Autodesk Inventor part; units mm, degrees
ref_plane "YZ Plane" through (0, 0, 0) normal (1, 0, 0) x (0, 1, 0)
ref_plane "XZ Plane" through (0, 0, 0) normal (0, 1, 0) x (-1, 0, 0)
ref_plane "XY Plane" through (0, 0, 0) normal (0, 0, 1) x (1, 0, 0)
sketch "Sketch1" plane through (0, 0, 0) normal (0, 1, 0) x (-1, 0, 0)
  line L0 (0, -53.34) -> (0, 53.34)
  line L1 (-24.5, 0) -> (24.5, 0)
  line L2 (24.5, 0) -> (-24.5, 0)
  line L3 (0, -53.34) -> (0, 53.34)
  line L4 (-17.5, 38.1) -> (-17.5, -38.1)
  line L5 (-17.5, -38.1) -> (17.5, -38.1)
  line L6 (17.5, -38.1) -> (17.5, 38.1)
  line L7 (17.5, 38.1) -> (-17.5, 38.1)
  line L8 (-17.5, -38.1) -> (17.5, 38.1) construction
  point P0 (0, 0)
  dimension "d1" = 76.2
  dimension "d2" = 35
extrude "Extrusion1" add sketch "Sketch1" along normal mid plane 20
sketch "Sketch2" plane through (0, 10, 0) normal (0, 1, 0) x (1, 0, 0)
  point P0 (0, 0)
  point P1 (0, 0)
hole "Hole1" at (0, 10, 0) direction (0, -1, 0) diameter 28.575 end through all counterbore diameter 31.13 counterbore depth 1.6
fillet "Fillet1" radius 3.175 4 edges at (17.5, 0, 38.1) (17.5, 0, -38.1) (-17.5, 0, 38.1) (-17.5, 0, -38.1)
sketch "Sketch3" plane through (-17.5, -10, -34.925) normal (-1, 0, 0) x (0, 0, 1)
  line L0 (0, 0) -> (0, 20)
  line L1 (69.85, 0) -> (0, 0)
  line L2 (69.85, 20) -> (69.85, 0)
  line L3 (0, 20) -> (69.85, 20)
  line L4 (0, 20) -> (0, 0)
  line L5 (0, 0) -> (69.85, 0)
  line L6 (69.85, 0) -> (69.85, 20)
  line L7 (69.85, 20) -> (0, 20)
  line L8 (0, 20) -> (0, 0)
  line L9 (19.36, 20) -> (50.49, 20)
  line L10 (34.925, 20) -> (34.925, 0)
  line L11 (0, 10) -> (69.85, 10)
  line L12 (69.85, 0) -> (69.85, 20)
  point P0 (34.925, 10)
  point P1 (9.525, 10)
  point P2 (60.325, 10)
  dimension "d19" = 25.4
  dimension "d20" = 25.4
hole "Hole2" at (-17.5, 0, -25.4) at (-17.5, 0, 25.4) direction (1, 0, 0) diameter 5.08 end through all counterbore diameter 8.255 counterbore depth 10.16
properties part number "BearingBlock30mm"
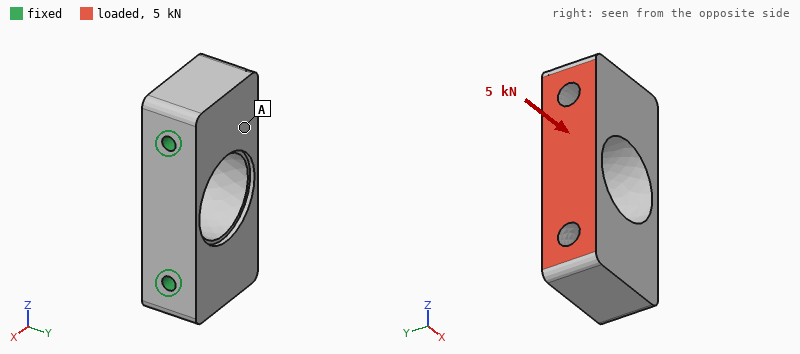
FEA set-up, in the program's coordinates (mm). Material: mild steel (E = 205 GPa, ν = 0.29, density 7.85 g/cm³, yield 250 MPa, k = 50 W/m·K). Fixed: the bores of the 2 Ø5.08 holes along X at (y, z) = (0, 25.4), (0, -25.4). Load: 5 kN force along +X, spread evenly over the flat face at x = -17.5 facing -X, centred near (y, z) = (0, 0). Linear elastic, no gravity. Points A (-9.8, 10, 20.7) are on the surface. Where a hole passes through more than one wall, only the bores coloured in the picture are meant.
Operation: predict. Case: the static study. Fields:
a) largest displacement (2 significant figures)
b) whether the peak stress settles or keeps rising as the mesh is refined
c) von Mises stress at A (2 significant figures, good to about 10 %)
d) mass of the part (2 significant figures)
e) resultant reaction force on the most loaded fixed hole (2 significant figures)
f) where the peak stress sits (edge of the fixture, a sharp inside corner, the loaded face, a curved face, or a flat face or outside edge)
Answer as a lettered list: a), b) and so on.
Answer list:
a) 4.1 µm
b) keeps rising
c) 3.3 MPa
d) 300 g
e) 2.6 kN
f) edge of the fixture
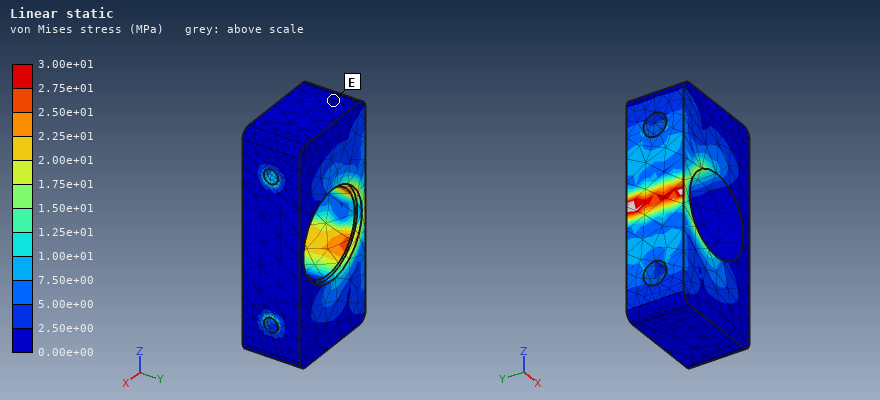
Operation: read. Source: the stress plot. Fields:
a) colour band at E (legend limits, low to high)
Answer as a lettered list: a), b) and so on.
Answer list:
a) 0.00e+00 to 2.50e+00 MPa
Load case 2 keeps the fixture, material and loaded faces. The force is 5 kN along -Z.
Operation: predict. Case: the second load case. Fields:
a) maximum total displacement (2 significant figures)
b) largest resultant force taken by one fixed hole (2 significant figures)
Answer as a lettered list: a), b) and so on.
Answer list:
a) 3.6 µm
b) 2.6 kN
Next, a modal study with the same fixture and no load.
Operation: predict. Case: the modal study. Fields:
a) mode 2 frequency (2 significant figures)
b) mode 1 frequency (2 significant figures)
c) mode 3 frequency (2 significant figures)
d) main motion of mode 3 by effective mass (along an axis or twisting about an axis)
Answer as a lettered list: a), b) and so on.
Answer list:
a) 22 kHz
b) 17 kHz
c) 23 kHz
d) along Z
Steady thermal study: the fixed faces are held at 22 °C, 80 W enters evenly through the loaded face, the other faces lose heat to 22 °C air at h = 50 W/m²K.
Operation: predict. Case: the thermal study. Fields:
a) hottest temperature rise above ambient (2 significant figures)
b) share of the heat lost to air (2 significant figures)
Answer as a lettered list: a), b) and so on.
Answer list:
a) 57 K
b) 6.8 %
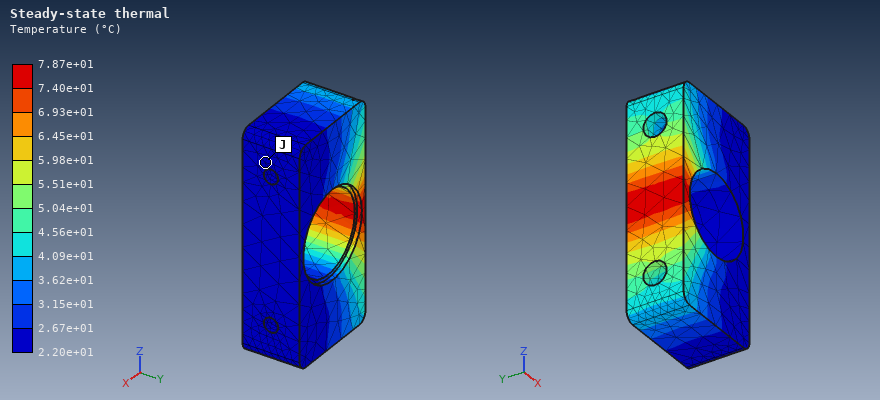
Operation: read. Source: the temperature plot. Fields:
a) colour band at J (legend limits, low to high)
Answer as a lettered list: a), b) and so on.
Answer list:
a) 2.20e+01 to 2.67e+01 °C
